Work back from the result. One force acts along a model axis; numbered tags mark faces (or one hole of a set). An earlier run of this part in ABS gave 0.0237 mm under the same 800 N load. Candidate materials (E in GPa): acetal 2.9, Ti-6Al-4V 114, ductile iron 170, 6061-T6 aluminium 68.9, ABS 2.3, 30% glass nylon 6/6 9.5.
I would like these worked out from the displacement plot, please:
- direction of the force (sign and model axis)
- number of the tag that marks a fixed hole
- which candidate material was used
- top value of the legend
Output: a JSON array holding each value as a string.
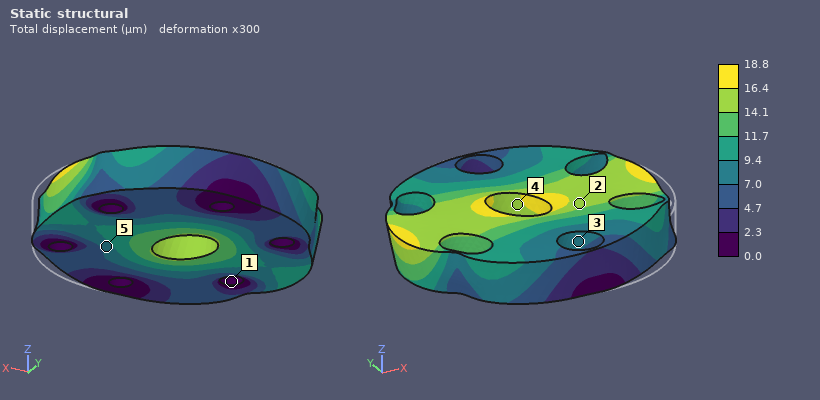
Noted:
["-X", "1", "acetal", "18.8 µm"]
